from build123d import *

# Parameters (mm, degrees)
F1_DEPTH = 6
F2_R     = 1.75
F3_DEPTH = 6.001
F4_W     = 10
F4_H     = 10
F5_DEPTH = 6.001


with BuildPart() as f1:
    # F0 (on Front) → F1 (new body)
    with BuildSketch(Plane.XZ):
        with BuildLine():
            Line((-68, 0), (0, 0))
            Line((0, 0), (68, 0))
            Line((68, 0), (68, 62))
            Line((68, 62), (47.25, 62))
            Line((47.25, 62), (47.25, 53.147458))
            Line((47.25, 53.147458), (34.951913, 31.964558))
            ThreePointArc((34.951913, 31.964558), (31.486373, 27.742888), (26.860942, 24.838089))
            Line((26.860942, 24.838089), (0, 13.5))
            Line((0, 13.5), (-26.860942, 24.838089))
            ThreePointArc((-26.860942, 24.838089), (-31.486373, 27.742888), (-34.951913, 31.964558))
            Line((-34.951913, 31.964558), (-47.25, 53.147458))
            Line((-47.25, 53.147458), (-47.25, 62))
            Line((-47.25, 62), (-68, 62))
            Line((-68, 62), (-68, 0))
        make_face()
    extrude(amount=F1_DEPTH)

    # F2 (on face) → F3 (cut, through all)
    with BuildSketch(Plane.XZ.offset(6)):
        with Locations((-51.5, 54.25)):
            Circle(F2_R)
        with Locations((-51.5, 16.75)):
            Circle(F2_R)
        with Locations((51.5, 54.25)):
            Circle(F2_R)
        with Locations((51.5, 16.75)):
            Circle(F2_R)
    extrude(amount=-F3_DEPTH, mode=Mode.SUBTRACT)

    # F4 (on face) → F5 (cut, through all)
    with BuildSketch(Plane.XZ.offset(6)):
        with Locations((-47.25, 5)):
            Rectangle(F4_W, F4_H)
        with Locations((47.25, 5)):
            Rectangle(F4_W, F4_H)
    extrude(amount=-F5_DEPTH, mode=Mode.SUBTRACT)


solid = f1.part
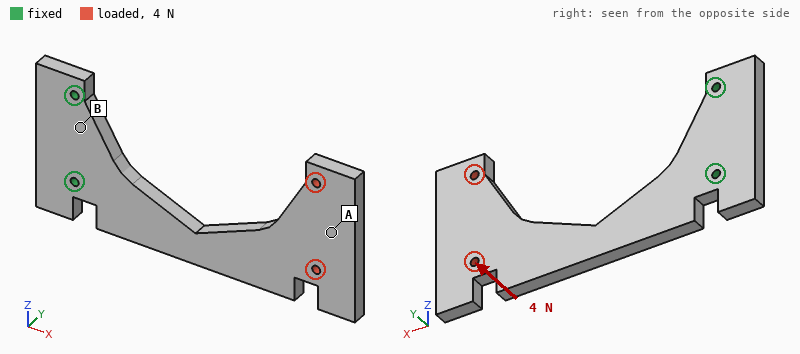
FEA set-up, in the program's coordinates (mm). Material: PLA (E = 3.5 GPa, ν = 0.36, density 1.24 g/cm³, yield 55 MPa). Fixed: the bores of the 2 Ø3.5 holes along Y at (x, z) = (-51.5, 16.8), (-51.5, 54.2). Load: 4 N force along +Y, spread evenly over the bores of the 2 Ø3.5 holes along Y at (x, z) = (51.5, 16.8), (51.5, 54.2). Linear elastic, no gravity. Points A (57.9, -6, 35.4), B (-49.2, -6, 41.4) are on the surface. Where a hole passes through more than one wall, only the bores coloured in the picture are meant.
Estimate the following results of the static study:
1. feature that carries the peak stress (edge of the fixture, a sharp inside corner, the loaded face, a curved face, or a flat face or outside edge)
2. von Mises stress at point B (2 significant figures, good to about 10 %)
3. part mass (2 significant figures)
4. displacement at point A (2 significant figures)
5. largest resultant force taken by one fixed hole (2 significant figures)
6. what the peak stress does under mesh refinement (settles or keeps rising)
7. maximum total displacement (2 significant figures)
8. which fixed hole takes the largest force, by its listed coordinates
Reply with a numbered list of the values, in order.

1. edge of the fixture
2. 0.83 MPa
3. 36 g
4. 1.4 mm
5. 4.1 N
6. keeps rising
7. 1.7 mm
8. (-51.5, 16.8)
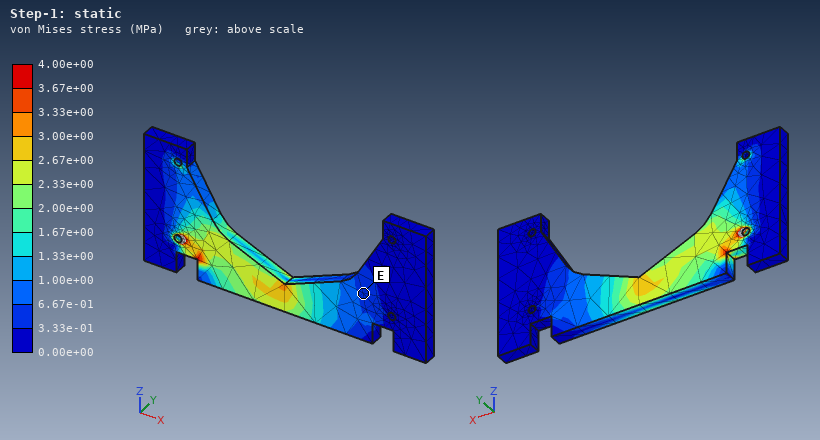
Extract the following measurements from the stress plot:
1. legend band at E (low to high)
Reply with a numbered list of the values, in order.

1. 3.33e-01 to 6.67e-01 MPa
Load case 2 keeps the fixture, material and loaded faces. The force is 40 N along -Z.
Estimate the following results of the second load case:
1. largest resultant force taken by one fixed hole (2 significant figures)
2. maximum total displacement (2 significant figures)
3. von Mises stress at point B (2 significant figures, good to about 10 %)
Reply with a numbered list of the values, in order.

1. 120 N
2. 1.6 mm
3. 1.6 MPa
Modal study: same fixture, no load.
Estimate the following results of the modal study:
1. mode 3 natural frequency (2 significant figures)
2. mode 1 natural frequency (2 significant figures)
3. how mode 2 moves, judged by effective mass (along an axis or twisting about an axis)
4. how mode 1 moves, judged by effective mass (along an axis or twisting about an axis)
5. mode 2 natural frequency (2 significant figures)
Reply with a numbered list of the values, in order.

1. 310 Hz
2. 74 Hz
3. along Z
4. along Y
5. 230 Hz
